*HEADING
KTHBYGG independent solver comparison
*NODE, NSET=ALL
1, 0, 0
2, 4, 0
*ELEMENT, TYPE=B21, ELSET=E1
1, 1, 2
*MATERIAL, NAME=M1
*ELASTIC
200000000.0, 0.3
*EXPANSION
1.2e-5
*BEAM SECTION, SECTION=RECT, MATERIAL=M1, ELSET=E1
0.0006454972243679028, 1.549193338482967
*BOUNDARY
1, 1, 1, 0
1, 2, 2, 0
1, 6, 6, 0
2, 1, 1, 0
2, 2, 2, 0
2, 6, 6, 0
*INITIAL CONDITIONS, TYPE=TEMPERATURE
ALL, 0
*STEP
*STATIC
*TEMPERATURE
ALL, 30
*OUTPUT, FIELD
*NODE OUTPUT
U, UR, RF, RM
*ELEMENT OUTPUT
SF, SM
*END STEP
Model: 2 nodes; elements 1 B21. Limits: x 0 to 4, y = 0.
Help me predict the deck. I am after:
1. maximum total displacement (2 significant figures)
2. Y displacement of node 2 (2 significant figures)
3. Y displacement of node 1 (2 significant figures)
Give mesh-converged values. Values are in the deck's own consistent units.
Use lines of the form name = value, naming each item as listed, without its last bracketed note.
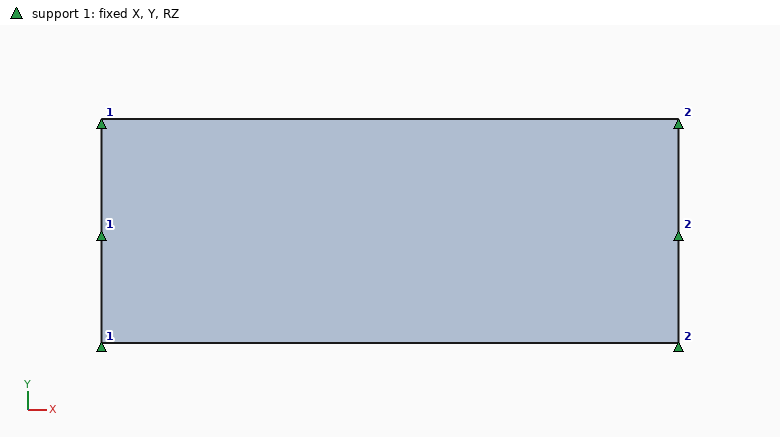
maximum total displacement = 3.6e-04
Y displacement of node 2 = 3.6e-04
Y displacement of node 1 = -3.6e-04
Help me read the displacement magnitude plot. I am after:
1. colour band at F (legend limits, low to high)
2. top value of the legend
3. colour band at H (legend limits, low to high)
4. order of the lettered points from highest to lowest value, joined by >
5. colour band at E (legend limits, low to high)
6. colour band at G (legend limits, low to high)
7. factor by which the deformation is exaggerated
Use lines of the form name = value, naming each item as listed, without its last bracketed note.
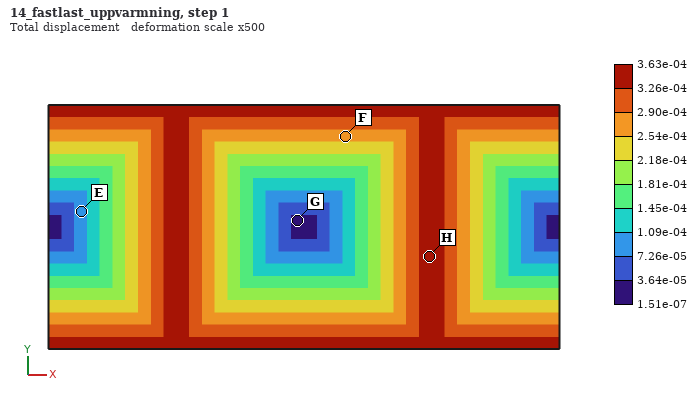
colour band at F = 2.54e-04 to 2.90e-04
top value of the legend = 3.63e-04
colour band at H = 3.26e-04 to 3.63e-04
order of the lettered points from highest to lowest value, joined by > = H > F > E > G
colour band at E = 7.26e-05 to 1.09e-04
colour band at G = 1.51e-07 to 3.64e-05
factor by which the deformation is exaggerated = 500
